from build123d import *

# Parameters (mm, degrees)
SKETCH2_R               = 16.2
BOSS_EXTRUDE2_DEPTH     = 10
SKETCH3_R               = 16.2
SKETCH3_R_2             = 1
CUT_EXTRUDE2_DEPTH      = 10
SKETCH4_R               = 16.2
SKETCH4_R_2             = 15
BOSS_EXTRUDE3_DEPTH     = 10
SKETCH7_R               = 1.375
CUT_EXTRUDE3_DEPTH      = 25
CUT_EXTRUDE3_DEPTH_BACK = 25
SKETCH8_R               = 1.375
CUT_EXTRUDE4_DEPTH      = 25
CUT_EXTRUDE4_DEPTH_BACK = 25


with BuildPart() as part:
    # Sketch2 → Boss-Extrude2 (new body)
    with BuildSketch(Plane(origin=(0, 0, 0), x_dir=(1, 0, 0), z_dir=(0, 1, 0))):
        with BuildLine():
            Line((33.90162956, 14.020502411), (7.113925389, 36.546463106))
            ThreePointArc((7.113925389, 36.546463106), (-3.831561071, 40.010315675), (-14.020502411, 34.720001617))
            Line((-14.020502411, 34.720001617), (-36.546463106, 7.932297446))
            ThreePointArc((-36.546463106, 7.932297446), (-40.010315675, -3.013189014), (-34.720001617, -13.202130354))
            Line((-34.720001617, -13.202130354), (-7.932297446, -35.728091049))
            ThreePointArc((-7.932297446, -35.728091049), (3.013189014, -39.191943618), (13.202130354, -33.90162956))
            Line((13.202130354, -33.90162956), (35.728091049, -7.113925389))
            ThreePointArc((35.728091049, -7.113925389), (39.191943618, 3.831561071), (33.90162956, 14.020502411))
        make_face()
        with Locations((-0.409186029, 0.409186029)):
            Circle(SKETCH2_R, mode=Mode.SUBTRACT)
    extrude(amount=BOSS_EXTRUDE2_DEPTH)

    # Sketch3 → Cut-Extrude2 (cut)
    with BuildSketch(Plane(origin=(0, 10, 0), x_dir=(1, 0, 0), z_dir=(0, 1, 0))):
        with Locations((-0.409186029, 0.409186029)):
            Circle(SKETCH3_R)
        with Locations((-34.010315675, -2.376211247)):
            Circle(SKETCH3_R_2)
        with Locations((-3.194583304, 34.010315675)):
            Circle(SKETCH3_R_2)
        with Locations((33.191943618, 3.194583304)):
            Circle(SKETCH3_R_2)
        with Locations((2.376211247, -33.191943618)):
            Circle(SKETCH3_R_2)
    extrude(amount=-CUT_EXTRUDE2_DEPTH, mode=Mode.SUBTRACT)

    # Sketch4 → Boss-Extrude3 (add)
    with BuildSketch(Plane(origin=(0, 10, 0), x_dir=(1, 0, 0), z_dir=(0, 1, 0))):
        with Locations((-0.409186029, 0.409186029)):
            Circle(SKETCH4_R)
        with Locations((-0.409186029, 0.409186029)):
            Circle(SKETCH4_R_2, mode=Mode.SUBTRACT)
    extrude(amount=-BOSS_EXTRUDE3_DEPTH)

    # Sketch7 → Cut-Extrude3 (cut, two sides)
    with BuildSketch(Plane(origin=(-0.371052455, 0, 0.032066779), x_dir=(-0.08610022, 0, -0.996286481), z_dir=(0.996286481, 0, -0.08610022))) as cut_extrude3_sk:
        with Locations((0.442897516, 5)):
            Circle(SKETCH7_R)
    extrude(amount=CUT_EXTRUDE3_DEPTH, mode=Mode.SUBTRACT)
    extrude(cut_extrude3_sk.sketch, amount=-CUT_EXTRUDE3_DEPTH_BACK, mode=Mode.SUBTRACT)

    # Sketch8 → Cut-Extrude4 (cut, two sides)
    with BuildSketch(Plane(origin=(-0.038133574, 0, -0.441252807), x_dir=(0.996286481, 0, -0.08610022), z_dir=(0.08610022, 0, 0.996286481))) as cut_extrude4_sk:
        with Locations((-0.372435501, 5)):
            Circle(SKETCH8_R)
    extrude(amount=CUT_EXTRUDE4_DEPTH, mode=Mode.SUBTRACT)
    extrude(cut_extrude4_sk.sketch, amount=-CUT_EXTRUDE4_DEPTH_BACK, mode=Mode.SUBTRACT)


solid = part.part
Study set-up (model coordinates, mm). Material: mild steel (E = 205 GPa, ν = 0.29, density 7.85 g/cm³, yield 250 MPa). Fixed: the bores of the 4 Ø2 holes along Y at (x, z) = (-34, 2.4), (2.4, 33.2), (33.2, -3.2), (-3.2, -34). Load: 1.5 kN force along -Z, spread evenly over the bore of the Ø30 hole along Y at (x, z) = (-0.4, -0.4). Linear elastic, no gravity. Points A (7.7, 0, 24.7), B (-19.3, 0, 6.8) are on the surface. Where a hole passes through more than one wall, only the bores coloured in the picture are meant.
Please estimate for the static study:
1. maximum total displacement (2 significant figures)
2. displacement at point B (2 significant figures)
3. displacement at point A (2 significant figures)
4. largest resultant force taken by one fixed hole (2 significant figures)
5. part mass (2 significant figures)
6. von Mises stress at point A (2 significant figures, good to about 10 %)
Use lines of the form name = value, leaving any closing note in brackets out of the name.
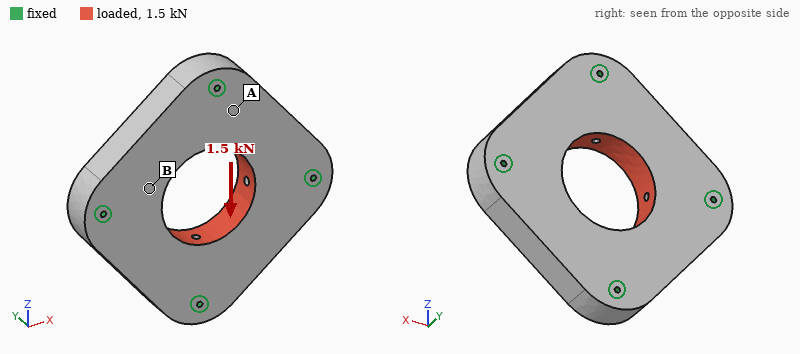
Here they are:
maximum total displacement = 0.47 µm
displacement at point B = 0.36 µm
displacement at point A = 0.21 µm
largest resultant force taken by one fixed hole = 470 N
part mass = 260 g
von Mises stress at point A = 2.7 MPa
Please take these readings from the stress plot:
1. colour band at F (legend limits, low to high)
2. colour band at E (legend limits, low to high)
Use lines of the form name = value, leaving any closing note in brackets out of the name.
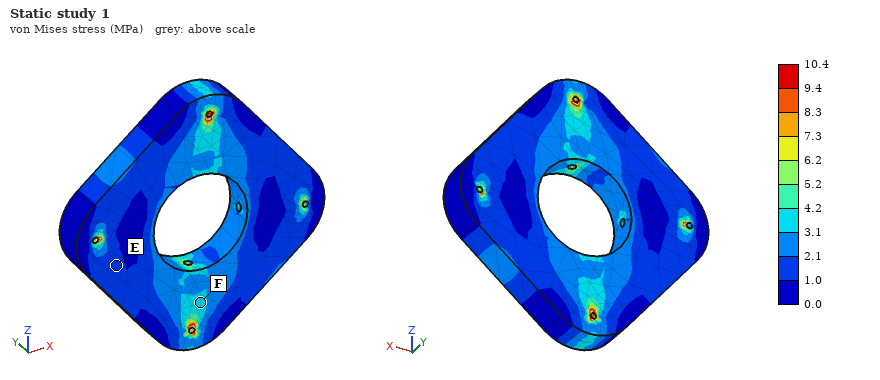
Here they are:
colour band at F = 3.1 to 4.2 MPa
colour band at E = 1.0 to 2.1 MPa
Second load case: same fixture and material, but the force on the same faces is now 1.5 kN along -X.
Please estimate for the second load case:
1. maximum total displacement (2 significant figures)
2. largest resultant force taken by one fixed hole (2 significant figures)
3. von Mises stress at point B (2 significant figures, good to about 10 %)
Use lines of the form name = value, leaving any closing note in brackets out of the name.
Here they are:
maximum total displacement = 0.47 µm
largest resultant force taken by one fixed hole = 470 N
von Mises stress at point B = 3.1 MPa
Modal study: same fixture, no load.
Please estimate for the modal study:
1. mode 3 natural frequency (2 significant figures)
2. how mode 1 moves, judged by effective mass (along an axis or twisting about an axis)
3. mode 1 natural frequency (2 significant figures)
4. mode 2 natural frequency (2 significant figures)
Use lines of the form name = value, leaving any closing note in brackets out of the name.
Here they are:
mode 3 natural frequency = 16 kHz
how mode 1 moves, judged by effective mass = along Y
mode 1 natural frequency = 13 kHz
mode 2 natural frequency = 16 kHz
